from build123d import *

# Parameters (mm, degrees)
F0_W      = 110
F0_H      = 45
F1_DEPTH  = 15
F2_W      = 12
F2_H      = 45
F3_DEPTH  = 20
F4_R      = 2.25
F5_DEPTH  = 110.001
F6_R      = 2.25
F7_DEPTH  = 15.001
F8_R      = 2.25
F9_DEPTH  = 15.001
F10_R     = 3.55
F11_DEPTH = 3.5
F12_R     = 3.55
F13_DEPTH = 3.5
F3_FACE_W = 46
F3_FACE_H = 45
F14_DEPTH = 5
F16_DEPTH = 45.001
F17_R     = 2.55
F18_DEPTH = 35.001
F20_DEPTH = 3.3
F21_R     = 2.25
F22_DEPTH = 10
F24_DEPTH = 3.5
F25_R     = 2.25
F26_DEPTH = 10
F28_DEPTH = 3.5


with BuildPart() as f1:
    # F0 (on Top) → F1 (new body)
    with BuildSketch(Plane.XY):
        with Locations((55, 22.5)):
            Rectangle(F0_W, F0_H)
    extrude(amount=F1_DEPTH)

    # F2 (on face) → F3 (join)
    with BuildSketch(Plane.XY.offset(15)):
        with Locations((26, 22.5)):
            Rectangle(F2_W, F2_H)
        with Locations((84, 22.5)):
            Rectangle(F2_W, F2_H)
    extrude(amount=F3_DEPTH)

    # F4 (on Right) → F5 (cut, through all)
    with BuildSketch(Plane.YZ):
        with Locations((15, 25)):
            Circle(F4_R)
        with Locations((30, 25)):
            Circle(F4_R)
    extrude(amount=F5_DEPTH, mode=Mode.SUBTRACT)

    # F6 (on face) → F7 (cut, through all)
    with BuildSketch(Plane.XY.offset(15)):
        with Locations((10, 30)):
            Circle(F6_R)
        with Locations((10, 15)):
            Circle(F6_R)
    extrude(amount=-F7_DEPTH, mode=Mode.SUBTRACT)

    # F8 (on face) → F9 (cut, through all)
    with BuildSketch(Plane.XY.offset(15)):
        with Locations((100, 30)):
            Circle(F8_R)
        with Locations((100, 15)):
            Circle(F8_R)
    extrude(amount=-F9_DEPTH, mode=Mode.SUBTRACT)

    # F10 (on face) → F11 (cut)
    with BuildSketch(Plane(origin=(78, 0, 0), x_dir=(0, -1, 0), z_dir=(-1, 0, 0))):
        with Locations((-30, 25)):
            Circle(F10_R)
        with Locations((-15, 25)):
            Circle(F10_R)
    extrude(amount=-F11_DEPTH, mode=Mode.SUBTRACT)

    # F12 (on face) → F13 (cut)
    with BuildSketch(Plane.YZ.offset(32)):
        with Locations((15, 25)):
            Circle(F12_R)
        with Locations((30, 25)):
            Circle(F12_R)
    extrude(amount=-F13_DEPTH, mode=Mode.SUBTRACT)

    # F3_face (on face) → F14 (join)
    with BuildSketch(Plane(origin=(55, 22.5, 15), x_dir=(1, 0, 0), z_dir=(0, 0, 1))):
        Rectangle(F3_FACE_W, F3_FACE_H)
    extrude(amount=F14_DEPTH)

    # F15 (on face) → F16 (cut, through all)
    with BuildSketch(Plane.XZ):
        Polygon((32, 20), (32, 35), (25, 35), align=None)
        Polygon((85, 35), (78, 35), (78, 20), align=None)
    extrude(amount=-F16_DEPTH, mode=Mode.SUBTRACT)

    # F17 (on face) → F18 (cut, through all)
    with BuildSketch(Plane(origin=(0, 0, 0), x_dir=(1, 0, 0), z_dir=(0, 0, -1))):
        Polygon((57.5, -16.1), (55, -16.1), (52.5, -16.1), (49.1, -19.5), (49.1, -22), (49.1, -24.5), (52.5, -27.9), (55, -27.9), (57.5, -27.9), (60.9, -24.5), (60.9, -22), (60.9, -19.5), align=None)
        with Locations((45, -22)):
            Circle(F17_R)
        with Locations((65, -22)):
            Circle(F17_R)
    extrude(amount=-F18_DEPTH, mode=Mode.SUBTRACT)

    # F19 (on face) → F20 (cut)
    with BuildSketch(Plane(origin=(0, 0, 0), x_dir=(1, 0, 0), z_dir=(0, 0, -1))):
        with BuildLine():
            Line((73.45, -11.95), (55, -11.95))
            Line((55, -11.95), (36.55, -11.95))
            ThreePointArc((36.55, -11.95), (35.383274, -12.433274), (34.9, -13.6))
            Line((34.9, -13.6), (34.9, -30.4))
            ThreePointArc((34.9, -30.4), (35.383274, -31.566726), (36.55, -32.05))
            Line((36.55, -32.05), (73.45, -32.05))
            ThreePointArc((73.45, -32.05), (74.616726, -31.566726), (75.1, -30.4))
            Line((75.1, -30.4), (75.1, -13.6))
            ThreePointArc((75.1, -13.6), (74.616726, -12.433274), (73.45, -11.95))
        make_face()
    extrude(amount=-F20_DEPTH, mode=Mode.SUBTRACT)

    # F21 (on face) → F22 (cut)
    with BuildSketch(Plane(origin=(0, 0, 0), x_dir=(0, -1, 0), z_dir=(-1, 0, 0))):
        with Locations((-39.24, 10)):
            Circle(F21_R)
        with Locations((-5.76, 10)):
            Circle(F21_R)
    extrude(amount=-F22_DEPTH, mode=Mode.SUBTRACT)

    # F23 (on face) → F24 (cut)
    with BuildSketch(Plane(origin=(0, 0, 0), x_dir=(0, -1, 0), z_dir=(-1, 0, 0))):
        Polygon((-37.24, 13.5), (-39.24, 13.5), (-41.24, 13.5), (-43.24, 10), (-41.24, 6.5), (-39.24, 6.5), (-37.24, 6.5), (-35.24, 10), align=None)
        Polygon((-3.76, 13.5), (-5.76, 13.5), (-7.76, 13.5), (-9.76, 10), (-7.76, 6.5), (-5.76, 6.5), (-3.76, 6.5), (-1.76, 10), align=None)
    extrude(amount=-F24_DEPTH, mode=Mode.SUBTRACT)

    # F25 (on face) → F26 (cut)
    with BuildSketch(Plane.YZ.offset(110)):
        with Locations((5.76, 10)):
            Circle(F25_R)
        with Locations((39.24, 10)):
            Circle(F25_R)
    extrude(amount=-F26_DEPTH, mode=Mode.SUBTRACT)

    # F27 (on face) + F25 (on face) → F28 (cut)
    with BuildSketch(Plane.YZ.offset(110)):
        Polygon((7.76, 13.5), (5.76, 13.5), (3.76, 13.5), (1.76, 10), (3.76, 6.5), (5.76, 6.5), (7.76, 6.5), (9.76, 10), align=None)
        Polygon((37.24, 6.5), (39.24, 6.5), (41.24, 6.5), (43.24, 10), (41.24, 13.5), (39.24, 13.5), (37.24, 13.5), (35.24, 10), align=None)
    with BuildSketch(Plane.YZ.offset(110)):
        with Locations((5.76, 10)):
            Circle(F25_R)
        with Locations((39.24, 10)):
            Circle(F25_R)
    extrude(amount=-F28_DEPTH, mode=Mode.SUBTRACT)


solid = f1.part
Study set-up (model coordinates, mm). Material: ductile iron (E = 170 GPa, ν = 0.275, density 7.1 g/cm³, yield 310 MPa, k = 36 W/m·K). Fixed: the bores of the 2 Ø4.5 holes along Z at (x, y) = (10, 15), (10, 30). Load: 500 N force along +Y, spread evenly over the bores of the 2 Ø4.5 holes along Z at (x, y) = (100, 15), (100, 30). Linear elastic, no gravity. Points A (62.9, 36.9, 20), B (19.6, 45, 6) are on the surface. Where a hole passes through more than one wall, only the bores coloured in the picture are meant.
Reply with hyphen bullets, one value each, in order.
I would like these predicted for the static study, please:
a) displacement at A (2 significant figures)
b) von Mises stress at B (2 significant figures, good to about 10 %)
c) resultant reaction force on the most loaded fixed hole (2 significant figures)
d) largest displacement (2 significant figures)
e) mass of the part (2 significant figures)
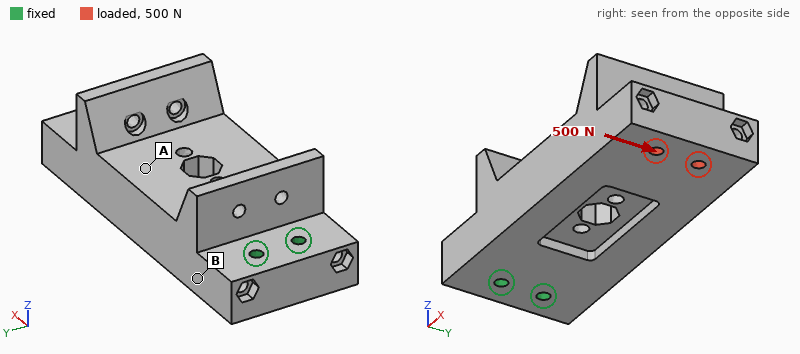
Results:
- 6.5 µm
- 4.7 MPa
- 2.4 kN
- 15 µm
- 660 g
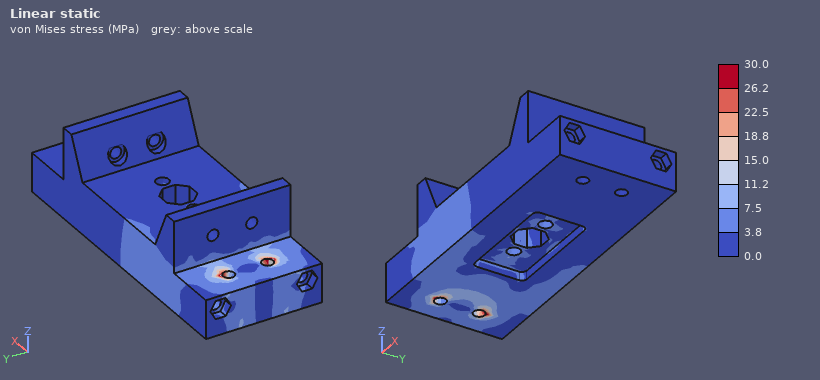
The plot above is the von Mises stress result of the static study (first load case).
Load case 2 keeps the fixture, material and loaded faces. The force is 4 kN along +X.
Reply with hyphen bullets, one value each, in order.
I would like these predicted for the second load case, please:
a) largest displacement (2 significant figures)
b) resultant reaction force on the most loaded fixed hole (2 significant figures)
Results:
- 12 µm
- 2.0 kN
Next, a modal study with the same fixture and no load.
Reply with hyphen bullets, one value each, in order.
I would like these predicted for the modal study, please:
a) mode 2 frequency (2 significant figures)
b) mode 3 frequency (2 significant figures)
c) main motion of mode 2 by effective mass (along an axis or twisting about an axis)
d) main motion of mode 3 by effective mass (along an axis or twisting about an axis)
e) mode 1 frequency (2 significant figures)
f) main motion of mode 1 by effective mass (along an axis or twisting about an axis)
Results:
- 2100 Hz
- 4100 Hz
- along Y
- twisting about X
- 1100 Hz
- along Z
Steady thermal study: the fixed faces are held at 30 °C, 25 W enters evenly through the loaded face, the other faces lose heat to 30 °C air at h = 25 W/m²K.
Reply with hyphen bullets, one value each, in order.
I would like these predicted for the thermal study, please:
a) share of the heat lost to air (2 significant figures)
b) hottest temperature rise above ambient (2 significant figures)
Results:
- 51 %
- 59 K
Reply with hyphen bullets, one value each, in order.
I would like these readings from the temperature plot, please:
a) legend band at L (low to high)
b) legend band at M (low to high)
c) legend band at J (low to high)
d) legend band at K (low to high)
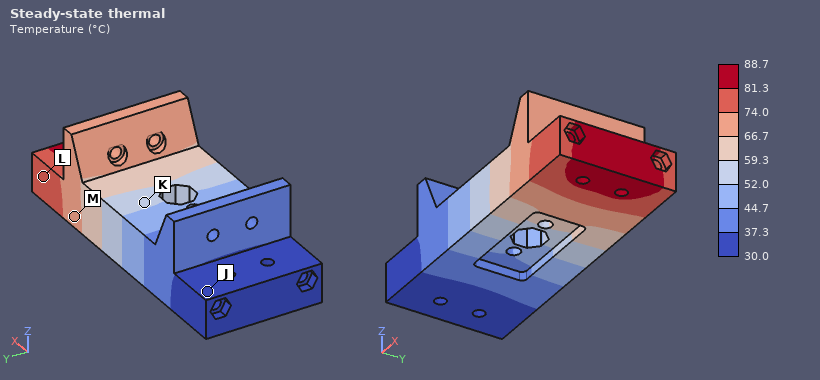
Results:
- 74.0 to 81.3 °C
- 66.7 to 74.0 °C
- 30.0 to 37.3 °C
- 52.0 to 59.3 °C
